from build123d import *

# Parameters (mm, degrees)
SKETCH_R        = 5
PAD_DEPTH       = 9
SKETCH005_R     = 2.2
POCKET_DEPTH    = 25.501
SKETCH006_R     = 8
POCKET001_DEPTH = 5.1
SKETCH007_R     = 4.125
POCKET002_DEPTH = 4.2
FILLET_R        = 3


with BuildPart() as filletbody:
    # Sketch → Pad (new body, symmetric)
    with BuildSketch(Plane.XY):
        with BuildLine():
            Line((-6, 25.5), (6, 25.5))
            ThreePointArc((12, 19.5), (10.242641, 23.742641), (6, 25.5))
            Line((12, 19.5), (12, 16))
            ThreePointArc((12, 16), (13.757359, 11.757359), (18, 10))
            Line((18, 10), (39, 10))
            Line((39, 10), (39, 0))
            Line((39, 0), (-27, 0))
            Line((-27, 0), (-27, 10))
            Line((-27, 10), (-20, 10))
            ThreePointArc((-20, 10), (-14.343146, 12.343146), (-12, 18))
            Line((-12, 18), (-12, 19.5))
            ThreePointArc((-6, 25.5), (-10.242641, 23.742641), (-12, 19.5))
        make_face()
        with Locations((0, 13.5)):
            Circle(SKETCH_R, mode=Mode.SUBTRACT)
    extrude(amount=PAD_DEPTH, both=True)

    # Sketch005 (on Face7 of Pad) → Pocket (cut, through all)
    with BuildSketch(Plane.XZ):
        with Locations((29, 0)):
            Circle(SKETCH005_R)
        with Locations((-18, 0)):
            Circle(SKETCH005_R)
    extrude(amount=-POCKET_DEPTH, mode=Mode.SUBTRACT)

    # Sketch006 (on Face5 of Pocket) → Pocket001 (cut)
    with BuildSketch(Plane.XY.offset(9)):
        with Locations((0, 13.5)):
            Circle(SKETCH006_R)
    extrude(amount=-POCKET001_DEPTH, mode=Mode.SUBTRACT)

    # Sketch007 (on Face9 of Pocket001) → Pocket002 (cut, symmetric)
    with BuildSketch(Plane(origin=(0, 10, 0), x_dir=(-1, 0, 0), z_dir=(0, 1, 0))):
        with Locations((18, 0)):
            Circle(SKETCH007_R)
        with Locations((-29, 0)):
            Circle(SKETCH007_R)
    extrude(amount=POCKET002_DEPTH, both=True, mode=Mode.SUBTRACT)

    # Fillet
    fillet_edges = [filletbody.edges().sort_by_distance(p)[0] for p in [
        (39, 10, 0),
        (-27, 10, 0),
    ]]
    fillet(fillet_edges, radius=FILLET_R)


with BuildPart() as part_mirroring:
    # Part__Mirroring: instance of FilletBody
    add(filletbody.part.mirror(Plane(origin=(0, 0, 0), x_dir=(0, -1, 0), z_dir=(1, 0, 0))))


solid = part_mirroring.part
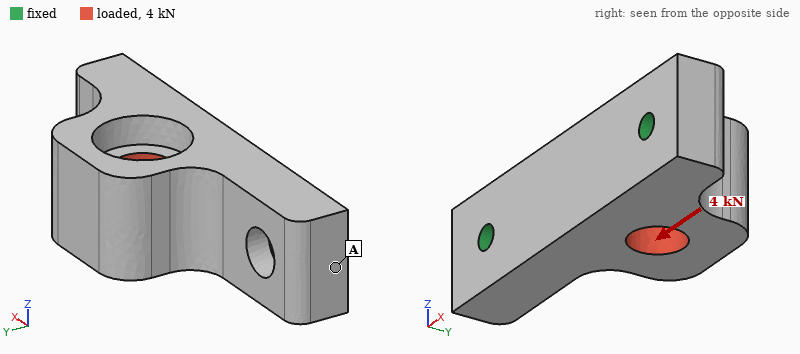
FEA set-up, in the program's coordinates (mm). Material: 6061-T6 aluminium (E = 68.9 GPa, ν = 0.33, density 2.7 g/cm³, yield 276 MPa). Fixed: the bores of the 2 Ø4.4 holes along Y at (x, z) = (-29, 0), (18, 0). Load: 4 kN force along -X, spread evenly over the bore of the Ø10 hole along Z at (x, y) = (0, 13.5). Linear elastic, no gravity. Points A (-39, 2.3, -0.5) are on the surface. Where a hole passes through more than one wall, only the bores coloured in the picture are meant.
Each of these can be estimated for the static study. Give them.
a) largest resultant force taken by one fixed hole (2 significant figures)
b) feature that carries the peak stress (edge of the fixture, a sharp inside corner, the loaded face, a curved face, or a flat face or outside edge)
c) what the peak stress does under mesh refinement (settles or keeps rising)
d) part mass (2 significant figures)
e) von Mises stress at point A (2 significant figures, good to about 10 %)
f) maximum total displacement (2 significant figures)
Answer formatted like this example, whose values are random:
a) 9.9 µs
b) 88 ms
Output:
a) 2.2 kN
b) edge of the fixture
c) keeps rising
d) 43 g
e) 8.0 MPa
f) 14 µm
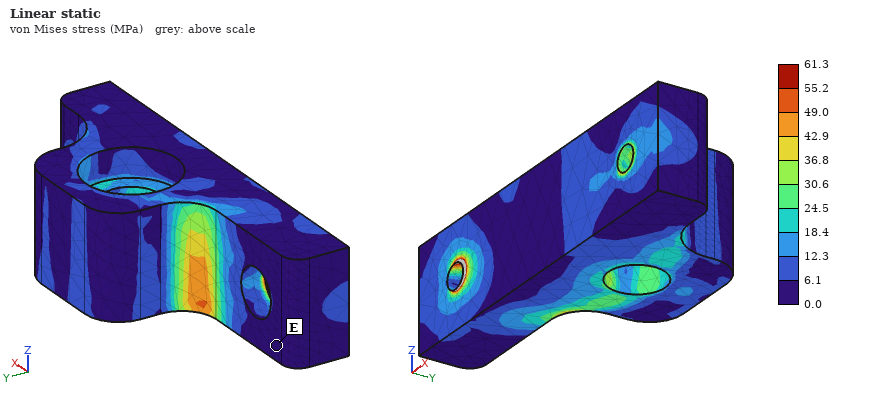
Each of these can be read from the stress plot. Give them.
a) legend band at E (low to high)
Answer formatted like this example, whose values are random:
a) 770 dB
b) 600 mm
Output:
a) 0.0 to 6.1 MPa
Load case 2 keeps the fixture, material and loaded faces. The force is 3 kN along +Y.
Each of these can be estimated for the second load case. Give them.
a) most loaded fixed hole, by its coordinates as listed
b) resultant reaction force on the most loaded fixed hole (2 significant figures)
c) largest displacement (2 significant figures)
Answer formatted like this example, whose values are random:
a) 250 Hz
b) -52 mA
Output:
a) (18, 0)
b) 2.1 kN
c) 29 µm
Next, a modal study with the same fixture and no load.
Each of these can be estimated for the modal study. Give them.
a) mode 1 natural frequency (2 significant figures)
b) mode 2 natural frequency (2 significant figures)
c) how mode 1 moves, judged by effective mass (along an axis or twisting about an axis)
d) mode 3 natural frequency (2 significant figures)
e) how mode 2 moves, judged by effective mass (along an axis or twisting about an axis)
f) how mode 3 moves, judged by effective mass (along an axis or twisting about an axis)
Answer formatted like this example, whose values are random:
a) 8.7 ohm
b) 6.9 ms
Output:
a) 7400 Hz
b) 13 kHz
c) along Z
d) 18 kHz
e) along Y
f) along Z
